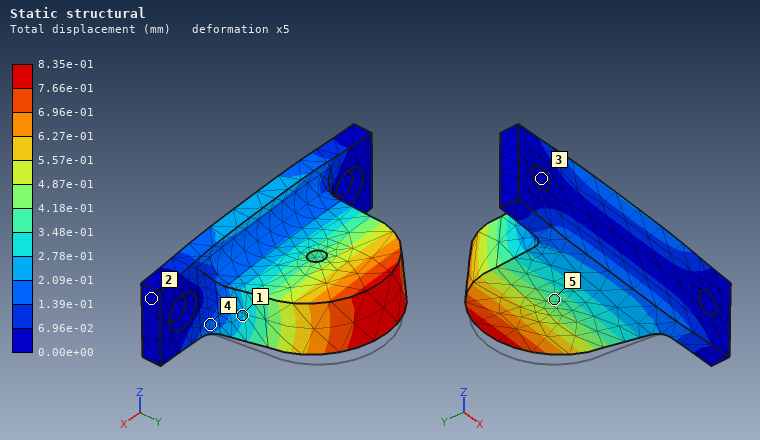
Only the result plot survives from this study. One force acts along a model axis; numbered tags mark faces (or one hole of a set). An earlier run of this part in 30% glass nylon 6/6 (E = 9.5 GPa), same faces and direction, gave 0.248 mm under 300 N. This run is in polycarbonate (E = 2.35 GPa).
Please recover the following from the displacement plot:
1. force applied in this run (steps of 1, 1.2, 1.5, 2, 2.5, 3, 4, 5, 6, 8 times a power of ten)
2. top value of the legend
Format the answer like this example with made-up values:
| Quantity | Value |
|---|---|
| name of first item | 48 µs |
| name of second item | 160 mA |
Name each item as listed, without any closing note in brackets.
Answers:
| Quantity | Value |
|---|---|
| force applied in this run | 250 N |
| top value of the legend | 8.35e-01 mm |
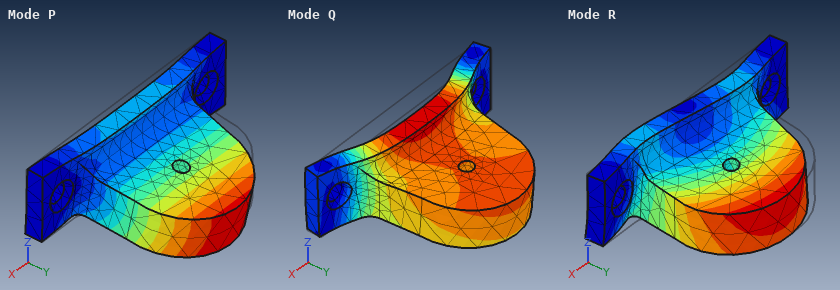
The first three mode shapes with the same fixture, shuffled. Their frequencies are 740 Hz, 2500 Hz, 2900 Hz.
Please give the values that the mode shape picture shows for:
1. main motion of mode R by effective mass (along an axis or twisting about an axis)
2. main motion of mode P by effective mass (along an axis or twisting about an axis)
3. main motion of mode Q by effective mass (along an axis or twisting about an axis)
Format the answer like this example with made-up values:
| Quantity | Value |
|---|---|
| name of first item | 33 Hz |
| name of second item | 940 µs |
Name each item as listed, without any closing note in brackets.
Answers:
| Quantity | Value |
|---|---|
| main motion of mode R by effective mass | along X |
| main motion of mode P by effective mass | along Z |
| main motion of mode Q by effective mass | along Y |
